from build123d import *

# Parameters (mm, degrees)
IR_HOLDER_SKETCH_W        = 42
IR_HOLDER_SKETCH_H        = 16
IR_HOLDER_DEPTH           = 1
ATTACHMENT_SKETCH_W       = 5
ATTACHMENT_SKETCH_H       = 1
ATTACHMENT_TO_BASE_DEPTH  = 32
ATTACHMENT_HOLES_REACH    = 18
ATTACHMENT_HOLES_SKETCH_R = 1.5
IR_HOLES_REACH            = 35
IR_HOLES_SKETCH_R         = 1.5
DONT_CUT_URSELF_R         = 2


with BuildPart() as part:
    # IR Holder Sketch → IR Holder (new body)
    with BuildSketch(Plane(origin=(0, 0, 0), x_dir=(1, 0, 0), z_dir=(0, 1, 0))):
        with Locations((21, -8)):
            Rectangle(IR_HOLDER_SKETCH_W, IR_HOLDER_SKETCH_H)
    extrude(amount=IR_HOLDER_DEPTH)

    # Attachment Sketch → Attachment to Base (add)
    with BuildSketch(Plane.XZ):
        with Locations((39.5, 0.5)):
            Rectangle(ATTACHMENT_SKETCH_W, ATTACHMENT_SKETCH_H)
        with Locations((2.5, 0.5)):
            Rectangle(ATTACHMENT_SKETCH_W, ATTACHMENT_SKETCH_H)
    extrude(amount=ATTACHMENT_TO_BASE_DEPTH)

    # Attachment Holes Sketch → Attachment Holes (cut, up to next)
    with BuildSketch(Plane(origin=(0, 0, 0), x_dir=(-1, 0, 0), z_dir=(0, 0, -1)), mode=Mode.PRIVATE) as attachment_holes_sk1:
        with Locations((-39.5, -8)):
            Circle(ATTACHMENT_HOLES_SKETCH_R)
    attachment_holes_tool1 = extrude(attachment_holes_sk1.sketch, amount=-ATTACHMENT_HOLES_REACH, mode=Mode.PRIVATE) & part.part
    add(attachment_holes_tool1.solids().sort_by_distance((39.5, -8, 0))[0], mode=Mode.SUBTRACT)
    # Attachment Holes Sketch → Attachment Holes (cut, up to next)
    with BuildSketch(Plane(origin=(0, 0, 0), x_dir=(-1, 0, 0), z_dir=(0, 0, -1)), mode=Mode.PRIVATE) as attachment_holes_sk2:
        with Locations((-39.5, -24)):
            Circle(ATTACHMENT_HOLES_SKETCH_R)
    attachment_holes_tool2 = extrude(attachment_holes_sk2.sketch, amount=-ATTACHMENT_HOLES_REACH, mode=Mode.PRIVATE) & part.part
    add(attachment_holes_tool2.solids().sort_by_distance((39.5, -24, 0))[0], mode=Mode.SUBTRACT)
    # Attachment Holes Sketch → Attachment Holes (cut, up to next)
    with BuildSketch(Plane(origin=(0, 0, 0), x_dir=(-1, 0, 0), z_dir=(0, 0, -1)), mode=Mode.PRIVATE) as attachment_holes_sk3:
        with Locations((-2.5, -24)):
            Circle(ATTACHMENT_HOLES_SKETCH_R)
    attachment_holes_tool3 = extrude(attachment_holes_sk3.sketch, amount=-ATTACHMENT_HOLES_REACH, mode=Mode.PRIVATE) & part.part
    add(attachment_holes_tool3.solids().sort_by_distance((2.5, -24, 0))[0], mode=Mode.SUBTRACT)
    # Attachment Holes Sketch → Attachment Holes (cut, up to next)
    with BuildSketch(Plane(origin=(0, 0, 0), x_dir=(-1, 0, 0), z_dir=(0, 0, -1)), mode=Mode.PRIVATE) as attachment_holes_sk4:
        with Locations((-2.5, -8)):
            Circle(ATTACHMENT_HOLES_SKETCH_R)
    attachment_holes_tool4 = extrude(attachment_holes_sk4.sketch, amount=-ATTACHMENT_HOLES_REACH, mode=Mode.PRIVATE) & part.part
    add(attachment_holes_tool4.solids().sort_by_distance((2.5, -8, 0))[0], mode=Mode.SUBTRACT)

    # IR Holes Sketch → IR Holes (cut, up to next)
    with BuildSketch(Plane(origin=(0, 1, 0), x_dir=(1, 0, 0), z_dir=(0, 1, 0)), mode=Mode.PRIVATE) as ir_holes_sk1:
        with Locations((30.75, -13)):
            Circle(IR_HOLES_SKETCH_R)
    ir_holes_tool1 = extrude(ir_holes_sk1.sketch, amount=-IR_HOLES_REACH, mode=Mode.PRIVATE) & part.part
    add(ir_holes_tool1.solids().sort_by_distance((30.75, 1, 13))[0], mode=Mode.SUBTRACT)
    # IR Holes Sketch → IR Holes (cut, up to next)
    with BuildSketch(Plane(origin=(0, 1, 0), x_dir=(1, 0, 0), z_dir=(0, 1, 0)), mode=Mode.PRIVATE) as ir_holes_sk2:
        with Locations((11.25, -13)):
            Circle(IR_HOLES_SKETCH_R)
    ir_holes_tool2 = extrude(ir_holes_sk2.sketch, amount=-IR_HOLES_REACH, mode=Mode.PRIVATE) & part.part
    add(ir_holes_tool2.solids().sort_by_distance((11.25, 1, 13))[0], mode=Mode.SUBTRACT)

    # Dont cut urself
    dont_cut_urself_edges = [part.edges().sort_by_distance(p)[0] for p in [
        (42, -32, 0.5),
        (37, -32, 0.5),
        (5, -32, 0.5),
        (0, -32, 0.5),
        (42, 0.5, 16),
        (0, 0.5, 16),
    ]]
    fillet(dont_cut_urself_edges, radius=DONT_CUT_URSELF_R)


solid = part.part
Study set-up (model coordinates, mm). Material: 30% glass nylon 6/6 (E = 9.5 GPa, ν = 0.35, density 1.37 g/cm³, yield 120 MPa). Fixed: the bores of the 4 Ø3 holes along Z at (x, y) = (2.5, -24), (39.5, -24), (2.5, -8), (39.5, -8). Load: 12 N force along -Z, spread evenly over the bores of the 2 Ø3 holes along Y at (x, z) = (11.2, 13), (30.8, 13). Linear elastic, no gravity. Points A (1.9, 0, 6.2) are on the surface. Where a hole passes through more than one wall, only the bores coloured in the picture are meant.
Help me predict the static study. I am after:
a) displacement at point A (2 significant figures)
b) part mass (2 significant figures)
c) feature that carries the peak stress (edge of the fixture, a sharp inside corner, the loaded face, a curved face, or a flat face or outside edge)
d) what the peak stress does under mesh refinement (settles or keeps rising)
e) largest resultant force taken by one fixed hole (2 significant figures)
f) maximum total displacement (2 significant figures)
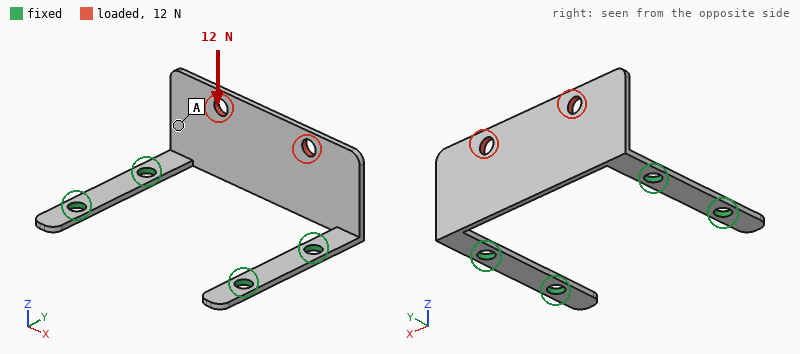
0.28 mm
1.3 g
edge of the fixture
keeps rising
6.0 N
0.64 mm
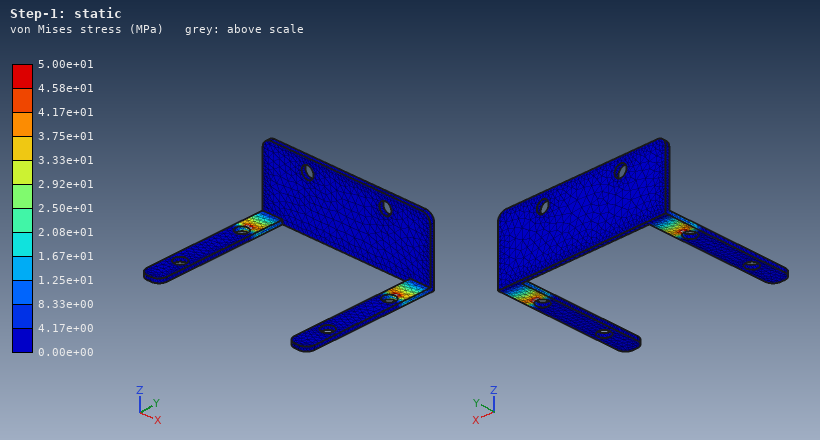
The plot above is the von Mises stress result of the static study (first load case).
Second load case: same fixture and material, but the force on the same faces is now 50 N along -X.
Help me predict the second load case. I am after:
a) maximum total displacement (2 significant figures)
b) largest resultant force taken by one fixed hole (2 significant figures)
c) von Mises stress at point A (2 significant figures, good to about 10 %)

0.66 mm
30 N
16 MPa
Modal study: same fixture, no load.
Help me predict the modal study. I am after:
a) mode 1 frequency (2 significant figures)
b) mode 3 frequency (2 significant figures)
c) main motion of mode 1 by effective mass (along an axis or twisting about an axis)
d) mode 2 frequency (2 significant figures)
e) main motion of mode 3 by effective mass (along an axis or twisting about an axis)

530 Hz
1900 Hz
along Y
1400 Hz
along Z
